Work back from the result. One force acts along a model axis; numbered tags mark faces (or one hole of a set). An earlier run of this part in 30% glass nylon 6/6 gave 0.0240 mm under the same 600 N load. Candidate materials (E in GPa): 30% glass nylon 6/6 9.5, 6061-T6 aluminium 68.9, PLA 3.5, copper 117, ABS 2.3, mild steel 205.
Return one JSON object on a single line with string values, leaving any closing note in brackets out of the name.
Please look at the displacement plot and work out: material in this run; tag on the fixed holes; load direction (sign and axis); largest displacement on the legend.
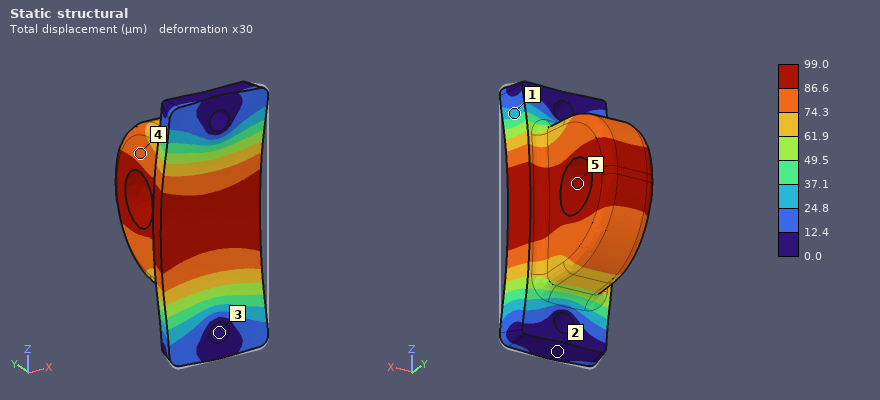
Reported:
{"material in this run": "ABS", "tag on the fixed holes": "3", "load direction": "+Y", "largest displacement on the legend": "99.0 µm"}
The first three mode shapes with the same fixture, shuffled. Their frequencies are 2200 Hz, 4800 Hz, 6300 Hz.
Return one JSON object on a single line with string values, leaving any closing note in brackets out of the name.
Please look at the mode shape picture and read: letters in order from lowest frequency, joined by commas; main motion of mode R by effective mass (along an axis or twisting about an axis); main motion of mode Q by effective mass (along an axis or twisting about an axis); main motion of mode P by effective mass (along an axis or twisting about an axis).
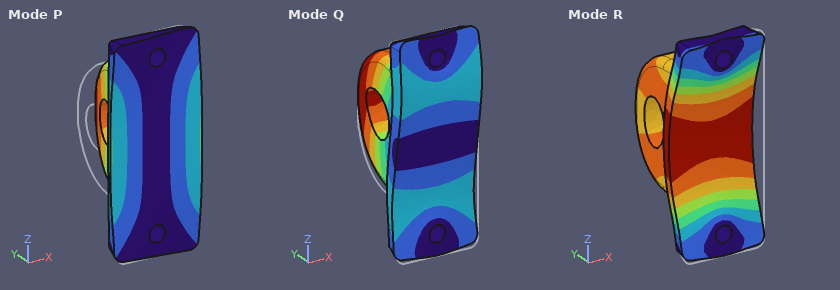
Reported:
{"letters in order from lowest frequency, joined by commas": "P, R, Q", "main motion of mode R by effective mass": "along Y", "main motion of mode Q by effective mass": "along Z", "main motion of mode P by effective mass": "along X"}
